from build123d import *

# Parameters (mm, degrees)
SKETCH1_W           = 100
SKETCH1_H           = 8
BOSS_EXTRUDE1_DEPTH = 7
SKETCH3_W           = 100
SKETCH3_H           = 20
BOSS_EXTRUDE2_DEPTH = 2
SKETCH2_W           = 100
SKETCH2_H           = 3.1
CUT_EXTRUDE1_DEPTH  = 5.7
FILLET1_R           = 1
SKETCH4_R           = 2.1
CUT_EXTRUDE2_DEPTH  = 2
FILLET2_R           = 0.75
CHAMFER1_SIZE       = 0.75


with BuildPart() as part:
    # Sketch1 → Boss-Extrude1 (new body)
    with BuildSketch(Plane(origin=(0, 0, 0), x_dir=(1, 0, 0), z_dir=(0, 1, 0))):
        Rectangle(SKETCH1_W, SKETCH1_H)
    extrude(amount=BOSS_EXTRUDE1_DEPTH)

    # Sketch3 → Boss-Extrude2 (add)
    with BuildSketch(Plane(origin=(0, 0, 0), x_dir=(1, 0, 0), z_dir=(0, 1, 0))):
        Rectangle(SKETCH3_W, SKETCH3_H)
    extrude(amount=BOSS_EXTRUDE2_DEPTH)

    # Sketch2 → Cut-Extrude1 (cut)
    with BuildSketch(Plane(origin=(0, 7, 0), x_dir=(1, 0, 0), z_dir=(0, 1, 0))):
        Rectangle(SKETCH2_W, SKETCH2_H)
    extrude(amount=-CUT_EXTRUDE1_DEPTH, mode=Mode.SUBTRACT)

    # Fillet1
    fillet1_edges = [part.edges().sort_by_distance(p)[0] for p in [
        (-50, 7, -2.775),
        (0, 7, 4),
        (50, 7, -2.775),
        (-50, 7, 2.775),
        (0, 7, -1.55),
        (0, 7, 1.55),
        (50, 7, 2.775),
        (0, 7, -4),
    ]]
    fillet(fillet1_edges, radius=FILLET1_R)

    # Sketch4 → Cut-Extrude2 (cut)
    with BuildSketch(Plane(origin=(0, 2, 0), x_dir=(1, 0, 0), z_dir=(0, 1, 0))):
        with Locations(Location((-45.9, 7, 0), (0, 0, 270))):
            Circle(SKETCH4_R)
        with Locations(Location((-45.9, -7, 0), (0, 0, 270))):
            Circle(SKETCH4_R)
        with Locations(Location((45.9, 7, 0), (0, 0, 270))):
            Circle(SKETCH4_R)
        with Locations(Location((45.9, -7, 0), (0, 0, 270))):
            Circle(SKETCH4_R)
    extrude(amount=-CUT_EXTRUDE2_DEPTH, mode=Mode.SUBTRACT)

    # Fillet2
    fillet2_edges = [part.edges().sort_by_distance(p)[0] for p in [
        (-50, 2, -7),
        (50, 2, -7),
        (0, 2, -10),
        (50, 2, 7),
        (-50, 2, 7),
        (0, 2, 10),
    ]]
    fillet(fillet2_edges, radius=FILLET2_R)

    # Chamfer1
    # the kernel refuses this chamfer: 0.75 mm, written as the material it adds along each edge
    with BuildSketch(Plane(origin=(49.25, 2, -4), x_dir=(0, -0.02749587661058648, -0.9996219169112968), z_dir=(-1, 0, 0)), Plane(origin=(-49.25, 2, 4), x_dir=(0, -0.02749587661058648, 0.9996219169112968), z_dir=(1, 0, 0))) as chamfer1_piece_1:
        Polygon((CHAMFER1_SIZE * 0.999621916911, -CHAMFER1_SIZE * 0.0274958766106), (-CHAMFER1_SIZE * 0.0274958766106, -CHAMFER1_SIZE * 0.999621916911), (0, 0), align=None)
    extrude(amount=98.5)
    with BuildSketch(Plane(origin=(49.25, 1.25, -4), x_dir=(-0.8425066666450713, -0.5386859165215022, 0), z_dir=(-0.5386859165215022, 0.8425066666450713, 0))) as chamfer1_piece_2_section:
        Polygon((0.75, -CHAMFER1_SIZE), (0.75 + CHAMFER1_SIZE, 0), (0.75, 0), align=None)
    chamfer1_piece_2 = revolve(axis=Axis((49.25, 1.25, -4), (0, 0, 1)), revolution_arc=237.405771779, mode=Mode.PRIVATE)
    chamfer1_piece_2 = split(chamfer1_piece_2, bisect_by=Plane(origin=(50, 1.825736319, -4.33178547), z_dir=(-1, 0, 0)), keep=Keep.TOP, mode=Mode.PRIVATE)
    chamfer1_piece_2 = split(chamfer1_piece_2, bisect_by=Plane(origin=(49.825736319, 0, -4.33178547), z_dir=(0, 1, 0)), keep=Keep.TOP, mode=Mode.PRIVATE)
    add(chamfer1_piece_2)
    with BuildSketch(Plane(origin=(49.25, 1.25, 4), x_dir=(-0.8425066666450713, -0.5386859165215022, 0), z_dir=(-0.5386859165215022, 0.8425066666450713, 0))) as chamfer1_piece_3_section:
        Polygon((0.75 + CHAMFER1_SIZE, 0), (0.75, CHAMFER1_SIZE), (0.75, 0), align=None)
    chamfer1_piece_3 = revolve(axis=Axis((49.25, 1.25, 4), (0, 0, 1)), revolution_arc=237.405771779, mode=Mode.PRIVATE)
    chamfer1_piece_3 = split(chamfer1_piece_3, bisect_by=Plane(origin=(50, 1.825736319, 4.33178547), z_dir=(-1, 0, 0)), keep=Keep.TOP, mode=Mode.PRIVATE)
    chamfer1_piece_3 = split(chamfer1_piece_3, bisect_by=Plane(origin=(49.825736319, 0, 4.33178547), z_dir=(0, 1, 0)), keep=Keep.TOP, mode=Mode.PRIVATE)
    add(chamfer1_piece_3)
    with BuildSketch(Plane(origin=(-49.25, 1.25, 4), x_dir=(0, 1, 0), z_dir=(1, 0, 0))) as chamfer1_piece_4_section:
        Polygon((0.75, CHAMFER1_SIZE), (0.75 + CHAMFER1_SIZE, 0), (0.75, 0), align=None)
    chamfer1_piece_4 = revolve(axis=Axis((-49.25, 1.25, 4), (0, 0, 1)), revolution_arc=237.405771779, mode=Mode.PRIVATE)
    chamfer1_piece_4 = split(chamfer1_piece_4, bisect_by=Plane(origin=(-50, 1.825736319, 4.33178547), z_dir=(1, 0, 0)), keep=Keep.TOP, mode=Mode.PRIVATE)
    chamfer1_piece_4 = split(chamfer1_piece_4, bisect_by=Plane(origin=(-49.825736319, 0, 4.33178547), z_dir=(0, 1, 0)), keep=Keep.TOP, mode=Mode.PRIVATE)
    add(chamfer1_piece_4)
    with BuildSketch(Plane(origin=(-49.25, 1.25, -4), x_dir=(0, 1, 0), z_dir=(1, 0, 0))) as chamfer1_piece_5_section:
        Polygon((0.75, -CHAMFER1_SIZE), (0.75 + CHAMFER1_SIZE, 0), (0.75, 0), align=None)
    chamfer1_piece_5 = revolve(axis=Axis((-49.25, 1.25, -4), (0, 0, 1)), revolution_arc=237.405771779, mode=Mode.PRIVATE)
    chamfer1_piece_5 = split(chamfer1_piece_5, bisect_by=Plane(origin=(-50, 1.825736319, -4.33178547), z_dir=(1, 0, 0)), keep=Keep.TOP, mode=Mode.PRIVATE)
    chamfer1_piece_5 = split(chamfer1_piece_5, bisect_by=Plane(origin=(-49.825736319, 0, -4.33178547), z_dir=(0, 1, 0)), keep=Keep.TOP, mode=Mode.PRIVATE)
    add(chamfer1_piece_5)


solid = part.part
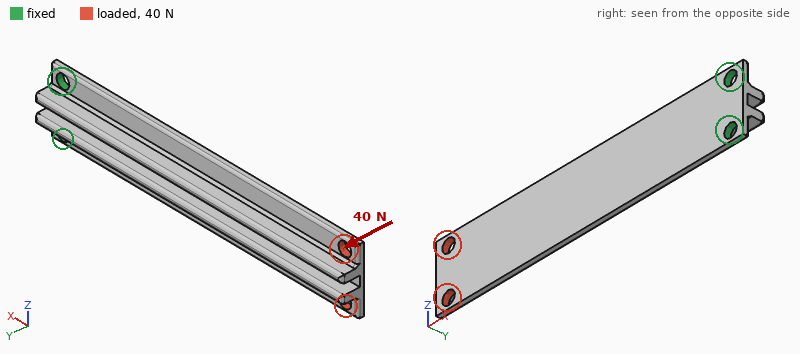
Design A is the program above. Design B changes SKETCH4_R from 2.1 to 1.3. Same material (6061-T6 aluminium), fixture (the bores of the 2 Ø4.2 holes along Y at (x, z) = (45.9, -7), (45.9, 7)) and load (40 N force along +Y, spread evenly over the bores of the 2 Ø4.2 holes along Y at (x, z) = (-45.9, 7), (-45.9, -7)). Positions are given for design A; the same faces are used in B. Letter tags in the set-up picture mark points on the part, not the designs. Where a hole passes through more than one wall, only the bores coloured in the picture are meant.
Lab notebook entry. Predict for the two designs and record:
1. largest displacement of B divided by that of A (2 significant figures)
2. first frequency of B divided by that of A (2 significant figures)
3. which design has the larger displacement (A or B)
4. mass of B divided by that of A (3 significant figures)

1.3
0.86
B
1.01
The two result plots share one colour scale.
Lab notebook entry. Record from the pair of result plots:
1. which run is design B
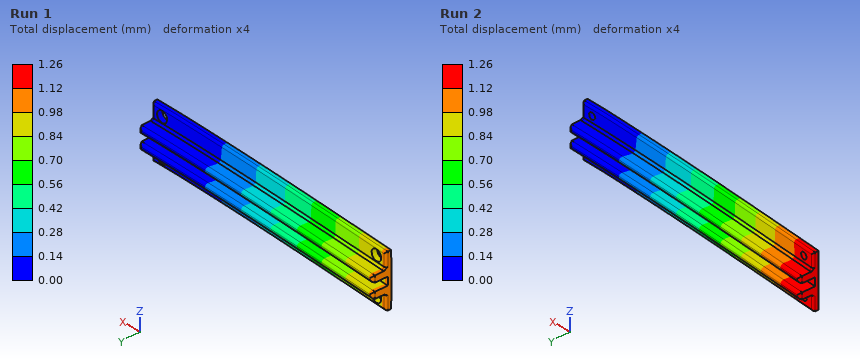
Run 2
